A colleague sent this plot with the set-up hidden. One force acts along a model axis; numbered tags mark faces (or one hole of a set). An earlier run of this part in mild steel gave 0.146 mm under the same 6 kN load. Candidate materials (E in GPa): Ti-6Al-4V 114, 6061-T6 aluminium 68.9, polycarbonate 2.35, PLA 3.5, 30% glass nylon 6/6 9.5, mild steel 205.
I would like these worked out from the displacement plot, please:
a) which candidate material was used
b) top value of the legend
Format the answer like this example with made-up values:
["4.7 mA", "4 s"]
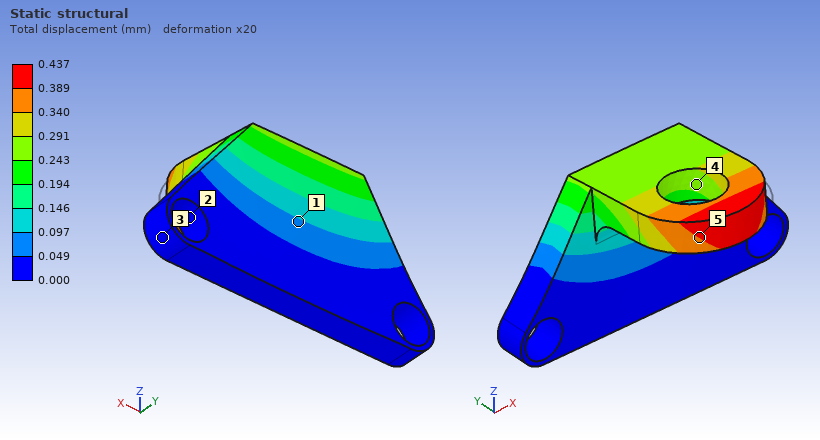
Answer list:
["6061-T6 aluminium", "0.437 mm"]
